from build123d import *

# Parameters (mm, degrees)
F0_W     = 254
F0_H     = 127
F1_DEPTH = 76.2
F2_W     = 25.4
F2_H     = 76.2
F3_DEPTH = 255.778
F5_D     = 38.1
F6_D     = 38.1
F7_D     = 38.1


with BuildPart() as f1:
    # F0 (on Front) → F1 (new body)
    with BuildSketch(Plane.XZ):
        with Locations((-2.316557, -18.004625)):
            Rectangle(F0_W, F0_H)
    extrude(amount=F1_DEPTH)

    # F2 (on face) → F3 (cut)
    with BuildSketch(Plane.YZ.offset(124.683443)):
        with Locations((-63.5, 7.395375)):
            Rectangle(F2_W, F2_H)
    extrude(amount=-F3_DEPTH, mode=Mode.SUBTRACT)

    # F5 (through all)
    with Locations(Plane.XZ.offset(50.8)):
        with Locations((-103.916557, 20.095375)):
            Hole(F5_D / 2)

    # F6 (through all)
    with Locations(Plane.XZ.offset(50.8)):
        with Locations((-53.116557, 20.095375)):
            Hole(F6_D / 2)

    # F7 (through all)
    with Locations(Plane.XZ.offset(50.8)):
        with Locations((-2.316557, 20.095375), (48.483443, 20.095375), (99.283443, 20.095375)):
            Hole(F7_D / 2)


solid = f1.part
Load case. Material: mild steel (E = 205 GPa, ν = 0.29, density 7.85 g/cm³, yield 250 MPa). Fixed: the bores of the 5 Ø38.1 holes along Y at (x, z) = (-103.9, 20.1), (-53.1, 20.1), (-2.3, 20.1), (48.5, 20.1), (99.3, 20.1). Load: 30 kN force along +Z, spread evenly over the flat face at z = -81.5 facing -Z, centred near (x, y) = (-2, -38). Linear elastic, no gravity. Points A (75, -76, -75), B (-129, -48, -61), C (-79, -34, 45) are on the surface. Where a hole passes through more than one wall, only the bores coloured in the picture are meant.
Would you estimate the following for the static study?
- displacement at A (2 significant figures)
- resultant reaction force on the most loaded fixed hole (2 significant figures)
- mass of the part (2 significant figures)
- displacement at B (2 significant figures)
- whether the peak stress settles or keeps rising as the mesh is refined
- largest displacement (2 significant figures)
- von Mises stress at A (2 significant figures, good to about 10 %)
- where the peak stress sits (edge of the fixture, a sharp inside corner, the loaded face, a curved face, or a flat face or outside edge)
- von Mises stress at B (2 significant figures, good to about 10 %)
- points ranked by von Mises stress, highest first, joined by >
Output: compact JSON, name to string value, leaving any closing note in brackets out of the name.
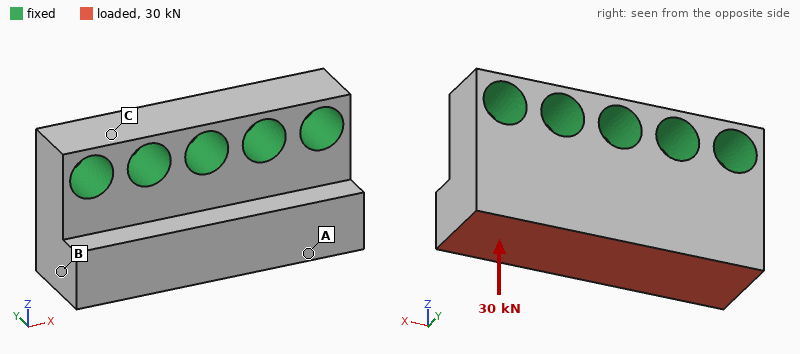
{"displacement at A": "3.3 µm", "resultant reaction force on the most loaded fixed hole": "6.6 kN", "mass of the part": "13 kg", "displacement at B": "2.0 µm", "whether the peak stress settles or keeps rising as the mesh is refined": "keeps rising", "largest displacement": "3.5 µm", "von Mises stress at A": "1.5 MPa", "where the peak stress sits": "edge of the fixture", "von Mises stress at B": "2.3 MPa", "points ranked by von Mises stress, highest first, joined by >": "B > A > C"}
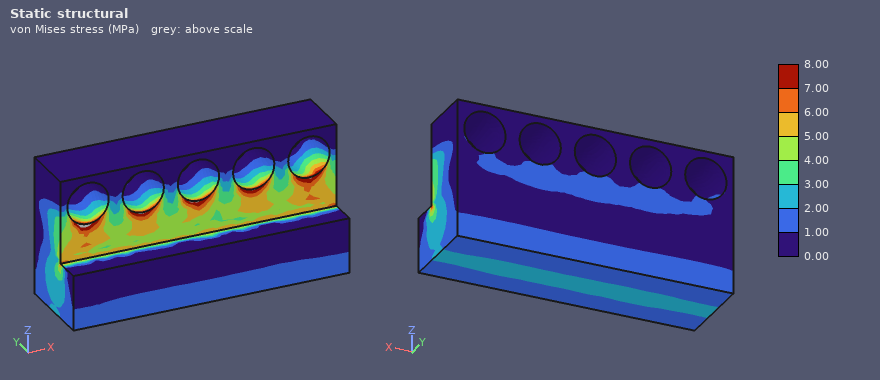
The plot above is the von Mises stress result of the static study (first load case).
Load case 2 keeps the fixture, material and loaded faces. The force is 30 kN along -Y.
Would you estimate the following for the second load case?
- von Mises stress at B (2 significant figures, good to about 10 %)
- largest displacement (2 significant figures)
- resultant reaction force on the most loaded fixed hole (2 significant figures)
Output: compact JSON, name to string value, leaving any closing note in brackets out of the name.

{"von Mises stress at B": "3.8 MPa", "largest displacement": "17 µm", "resultant reaction force on the most loaded fixed hole": "6.4 kN"}
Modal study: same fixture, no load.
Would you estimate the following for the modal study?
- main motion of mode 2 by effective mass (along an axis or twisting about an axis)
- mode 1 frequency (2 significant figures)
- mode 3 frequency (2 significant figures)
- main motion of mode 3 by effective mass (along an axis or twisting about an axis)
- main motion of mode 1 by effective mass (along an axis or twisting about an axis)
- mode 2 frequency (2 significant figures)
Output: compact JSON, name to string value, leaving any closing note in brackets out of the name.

{"main motion of mode 2 by effective mass": "twisting about Z", "mode 1 frequency": "3600 Hz", "mode 3 frequency": "6700 Hz", "main motion of mode 3 by effective mass": "along X", "main motion of mode 1 by effective mass": "along Y", "mode 2 frequency": "4600 Hz"}
